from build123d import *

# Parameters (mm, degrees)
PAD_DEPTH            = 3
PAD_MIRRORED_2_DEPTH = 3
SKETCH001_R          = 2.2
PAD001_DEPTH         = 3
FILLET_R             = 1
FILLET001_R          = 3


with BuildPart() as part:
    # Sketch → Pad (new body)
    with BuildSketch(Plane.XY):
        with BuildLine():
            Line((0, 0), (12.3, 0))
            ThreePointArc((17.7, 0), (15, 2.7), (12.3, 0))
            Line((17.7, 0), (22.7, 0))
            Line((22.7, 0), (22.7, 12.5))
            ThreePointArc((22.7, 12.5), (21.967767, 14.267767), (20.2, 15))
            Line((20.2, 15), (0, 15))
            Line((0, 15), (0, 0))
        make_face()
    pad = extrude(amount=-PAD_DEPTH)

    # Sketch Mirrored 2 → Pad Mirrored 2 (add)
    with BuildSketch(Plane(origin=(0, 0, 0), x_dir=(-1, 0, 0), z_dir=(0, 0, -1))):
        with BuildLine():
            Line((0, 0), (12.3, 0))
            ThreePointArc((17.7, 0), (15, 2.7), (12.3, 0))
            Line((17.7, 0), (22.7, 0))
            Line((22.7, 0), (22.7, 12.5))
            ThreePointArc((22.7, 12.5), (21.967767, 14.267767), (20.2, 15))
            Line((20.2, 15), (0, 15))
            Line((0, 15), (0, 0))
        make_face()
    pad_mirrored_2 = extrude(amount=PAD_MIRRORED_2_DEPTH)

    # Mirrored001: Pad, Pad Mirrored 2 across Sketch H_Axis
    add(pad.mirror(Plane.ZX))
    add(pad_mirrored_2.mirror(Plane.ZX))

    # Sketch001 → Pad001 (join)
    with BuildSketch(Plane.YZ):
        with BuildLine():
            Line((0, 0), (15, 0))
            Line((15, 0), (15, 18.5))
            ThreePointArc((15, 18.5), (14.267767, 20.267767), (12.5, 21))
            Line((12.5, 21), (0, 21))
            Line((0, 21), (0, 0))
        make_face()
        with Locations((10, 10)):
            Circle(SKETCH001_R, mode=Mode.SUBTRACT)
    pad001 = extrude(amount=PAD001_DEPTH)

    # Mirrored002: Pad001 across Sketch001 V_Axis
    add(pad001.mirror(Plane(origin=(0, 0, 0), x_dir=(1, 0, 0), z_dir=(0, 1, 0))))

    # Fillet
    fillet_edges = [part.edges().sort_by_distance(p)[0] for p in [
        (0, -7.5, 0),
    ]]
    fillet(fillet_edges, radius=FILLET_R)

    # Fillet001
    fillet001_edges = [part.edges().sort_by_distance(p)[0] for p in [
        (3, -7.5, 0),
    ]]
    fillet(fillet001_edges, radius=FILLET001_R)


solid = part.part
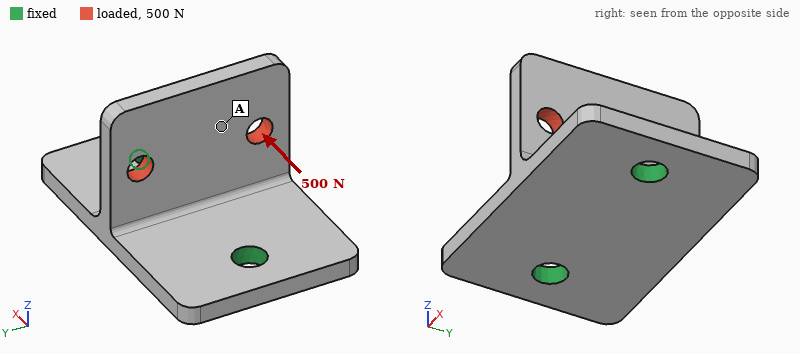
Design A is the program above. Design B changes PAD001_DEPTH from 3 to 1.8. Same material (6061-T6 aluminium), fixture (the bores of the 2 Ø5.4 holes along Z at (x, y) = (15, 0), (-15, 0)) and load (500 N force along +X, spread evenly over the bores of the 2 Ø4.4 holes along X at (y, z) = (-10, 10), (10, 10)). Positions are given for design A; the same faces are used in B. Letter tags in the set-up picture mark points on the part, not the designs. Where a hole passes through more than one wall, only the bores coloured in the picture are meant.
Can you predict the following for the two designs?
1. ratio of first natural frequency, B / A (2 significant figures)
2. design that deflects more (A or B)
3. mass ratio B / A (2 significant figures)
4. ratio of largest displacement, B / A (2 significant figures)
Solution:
0.71
B
0.88
3.0
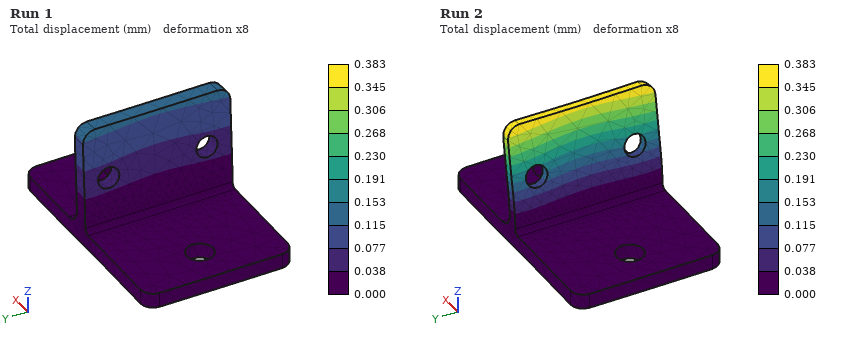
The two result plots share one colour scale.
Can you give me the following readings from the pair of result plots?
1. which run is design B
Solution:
Run 2
